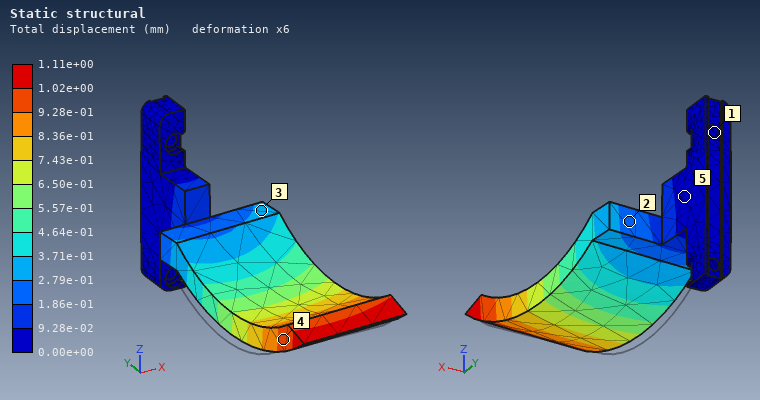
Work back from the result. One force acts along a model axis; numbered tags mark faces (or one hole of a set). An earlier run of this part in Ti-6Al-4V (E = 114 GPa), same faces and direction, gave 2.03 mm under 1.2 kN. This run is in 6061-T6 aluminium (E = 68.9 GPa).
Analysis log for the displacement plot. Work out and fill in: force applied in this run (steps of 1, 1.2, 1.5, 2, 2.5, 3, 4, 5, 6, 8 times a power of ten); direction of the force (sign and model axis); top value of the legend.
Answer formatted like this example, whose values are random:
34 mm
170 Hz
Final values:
400 N
+X
1.11e+00 mm
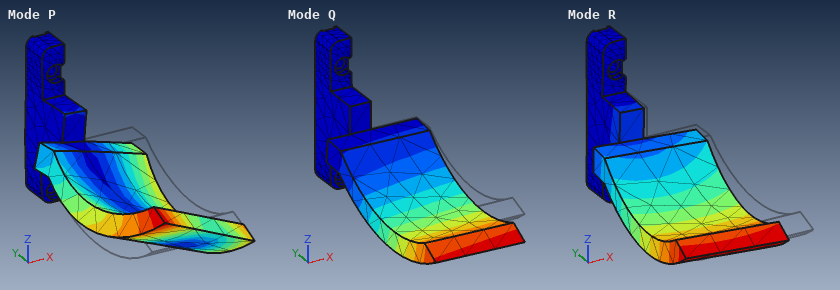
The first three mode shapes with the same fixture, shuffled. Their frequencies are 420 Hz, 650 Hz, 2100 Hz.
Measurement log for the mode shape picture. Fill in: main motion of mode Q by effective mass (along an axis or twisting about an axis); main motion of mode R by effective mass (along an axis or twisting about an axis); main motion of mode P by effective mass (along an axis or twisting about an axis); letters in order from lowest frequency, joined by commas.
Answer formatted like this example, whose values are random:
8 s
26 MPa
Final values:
along Z
along X
twisting about Y
R, Q, P
